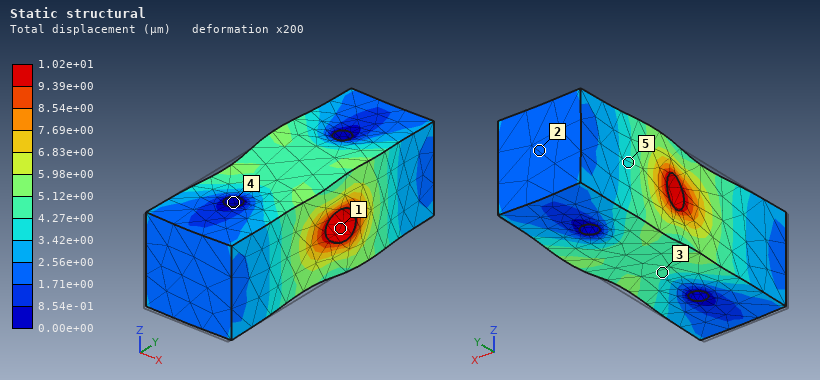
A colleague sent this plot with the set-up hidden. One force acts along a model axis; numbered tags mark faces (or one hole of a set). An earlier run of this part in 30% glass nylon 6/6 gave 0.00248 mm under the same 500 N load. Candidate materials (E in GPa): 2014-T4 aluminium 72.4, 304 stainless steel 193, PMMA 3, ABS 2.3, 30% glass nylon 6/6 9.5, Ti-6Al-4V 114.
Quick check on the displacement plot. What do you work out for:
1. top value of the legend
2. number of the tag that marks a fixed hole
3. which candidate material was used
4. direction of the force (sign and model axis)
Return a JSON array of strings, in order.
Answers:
["1.02e+01 µm", "4", "ABS", "+Y"]
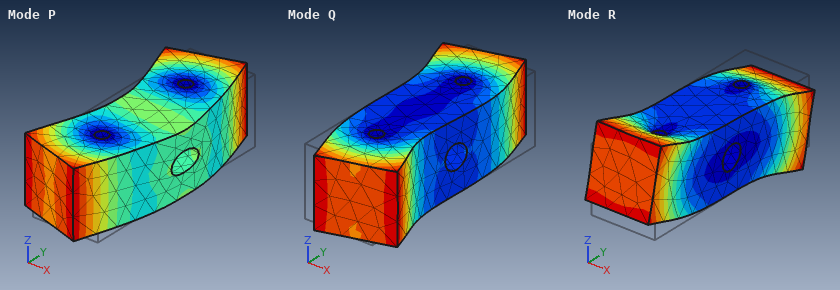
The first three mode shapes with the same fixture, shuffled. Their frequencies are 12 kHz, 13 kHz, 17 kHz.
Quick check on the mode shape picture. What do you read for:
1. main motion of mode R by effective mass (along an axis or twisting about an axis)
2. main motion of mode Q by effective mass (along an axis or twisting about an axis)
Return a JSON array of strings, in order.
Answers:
["twisting about X", "twisting about Z"]
